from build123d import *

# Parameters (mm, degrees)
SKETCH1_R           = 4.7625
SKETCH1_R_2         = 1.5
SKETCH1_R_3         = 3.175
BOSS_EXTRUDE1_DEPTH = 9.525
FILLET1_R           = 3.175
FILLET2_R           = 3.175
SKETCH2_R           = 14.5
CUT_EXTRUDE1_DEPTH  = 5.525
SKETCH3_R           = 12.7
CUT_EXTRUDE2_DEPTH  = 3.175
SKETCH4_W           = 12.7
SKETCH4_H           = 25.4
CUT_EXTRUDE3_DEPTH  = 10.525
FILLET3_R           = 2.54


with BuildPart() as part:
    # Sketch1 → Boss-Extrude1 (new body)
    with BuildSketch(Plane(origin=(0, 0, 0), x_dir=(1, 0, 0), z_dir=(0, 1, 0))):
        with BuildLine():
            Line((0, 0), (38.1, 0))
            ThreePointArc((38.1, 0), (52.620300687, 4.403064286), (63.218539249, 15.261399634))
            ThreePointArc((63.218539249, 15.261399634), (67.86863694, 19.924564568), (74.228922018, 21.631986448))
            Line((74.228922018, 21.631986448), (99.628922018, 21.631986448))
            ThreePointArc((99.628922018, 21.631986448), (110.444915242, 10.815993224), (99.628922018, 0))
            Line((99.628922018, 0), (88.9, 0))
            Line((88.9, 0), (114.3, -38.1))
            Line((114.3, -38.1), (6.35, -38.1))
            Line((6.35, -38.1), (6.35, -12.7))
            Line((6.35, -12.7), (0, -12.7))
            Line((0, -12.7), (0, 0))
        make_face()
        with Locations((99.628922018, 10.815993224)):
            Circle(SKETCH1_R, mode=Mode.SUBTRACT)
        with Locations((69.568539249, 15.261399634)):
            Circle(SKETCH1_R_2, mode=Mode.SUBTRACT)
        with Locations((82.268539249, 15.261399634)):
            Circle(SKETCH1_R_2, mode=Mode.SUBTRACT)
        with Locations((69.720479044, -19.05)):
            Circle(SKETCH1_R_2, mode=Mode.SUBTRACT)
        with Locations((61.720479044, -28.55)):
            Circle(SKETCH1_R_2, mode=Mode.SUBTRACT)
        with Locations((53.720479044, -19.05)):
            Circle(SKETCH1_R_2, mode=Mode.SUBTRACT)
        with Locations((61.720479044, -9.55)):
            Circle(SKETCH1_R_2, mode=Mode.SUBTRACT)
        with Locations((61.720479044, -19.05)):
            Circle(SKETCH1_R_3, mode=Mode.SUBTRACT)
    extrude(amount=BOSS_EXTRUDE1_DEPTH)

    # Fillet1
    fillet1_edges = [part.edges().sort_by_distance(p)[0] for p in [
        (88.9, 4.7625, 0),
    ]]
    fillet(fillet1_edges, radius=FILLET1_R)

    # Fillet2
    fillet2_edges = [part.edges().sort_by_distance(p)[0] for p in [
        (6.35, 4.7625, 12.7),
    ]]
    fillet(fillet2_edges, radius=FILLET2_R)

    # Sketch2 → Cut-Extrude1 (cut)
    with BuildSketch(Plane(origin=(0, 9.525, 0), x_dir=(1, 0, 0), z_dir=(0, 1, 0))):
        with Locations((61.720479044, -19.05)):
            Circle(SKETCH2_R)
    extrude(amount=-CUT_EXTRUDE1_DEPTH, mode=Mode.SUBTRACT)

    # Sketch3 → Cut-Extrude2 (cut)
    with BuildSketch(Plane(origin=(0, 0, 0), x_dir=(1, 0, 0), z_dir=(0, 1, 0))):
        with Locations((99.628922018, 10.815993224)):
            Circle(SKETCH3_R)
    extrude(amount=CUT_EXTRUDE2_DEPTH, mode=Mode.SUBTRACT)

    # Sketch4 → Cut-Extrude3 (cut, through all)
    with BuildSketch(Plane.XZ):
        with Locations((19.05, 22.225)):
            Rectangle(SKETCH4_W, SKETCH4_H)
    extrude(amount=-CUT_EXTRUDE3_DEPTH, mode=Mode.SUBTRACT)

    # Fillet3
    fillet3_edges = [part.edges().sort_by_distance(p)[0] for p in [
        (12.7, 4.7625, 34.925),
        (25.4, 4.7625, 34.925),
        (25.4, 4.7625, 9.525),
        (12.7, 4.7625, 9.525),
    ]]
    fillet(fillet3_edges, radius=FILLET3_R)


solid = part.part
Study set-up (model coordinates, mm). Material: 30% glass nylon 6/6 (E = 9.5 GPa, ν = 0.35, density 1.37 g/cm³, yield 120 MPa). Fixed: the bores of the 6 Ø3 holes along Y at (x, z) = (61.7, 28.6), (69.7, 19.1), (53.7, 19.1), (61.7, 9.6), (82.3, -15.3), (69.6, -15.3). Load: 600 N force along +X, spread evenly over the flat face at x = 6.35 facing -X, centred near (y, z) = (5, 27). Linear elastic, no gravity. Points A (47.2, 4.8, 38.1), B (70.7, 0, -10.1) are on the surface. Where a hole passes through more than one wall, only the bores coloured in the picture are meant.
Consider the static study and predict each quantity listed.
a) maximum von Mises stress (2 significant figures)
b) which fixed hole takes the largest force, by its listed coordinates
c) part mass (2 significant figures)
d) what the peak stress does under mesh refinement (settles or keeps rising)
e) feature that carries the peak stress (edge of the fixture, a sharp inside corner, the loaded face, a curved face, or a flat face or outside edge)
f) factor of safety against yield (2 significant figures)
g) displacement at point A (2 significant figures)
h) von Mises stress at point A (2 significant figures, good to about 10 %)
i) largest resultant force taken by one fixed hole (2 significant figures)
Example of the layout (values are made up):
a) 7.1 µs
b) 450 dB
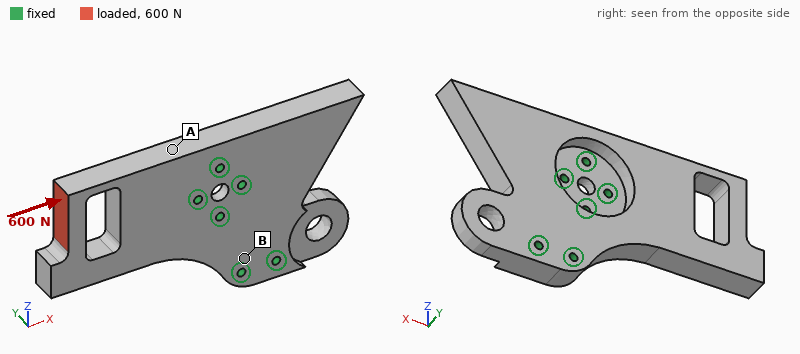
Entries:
a) 42 MPa
b) (61.7, 28.6)
c) 50 g
d) settles
e) a curved face
f) 2.9
g) 0.025 mm
h) 5.3 MPa
i) 330 N
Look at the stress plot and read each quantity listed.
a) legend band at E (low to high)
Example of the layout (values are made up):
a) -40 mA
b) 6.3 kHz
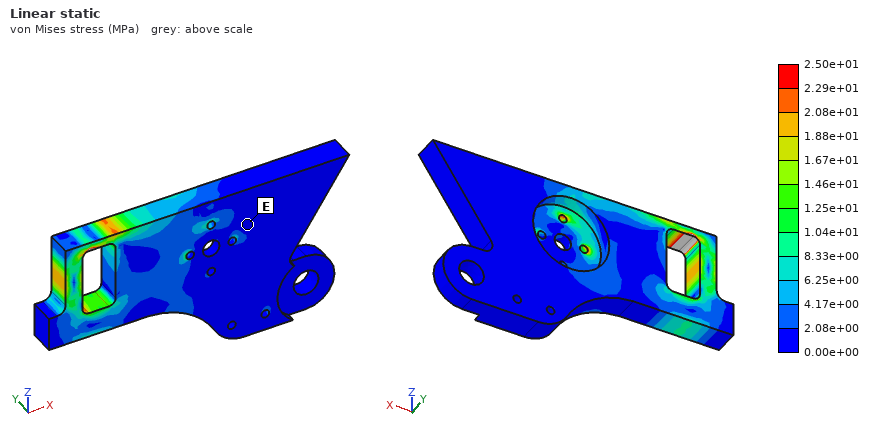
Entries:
a) 0.00e+00 to 2.08e+00 MPa
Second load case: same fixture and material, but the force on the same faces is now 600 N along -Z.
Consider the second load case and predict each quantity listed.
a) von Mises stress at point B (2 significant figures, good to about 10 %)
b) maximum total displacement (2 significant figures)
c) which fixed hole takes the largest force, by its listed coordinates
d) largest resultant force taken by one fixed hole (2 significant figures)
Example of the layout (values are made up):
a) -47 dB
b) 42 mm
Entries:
a) 4.1 MPa
b) 0.32 mm
c) (61.7, 28.6)
d) 690 N
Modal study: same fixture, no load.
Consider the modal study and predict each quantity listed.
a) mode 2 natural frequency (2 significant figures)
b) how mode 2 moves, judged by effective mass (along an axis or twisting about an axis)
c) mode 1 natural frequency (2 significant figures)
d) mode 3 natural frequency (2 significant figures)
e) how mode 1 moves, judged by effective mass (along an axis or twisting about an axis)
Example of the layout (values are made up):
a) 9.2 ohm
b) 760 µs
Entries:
a) 2000 Hz
b) along Y
c) 1100 Hz
d) 2800 Hz
e) along Y
